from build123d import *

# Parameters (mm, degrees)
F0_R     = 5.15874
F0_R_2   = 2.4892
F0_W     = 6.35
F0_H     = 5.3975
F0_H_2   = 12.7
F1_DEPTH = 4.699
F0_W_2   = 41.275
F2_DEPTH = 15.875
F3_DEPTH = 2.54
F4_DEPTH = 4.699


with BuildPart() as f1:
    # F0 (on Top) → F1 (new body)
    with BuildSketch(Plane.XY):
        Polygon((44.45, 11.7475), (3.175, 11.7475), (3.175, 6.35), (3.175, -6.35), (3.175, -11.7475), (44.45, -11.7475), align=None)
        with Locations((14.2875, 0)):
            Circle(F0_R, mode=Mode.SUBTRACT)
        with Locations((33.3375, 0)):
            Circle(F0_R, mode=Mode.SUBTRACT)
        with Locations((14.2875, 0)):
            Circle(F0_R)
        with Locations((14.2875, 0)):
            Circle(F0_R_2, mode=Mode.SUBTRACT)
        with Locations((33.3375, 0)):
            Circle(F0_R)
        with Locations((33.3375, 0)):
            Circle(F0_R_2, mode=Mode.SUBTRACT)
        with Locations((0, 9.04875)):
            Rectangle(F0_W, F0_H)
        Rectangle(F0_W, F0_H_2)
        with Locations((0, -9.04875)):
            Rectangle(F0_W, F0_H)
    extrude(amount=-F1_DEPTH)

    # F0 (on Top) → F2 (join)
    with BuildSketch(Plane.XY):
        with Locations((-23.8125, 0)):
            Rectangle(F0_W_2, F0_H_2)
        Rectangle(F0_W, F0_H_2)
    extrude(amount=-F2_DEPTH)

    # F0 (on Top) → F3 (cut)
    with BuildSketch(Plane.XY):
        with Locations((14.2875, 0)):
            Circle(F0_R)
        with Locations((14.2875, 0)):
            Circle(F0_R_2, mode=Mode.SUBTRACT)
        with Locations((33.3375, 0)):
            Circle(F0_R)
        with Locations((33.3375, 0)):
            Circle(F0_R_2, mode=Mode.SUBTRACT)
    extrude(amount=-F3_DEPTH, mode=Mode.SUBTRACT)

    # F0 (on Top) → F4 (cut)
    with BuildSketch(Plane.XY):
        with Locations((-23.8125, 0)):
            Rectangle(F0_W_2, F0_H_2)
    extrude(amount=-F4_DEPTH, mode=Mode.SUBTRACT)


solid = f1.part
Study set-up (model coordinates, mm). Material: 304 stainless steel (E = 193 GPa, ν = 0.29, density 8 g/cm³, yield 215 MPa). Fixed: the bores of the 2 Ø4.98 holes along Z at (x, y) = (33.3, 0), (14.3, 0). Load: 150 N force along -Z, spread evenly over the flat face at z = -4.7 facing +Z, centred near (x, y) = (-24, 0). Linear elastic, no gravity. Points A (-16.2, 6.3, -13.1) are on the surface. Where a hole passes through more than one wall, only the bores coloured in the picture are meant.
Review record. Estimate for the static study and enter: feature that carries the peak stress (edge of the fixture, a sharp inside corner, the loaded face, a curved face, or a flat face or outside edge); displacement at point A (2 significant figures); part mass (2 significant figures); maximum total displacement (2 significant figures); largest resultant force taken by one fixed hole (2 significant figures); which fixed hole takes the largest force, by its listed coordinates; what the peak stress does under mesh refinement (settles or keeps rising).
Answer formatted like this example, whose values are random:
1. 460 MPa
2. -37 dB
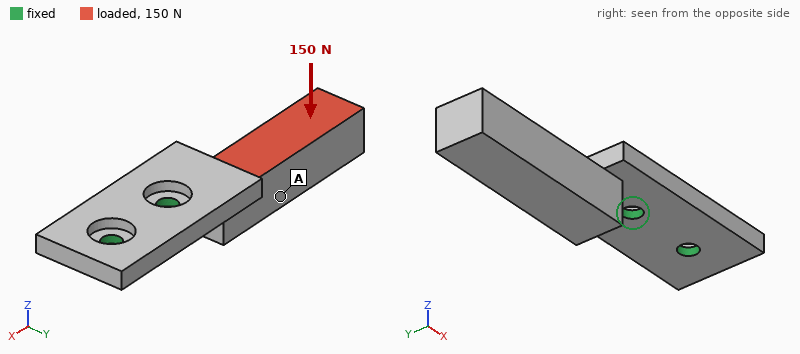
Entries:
1. edge of the fixture
2. 0.072 mm
3. 92 g
4. 0.15 mm
5. 550 N
6. (14.3, 0)
7. keeps rising
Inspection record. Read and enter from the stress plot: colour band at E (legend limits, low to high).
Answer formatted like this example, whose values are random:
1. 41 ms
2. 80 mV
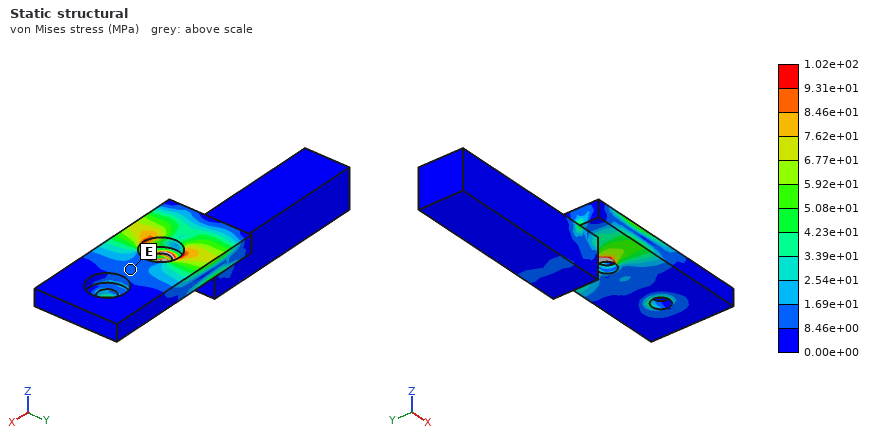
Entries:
1. 8.46e+00 to 1.69e+01 MPa
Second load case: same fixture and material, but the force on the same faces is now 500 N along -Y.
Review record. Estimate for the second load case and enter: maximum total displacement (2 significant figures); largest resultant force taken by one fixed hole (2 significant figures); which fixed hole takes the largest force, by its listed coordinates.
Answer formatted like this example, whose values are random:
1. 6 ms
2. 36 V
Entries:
1. 71 µm
2. 1.3 kN
3. (14.3, 0)
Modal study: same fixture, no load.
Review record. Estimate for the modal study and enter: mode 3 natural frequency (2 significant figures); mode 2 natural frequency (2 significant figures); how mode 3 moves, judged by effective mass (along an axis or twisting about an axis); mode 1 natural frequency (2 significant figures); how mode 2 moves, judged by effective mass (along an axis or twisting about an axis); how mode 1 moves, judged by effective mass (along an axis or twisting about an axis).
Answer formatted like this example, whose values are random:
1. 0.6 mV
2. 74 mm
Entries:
1. 5000 Hz
2. 2300 Hz
3. twisting about X
4. 860 Hz
5. along Y
6. along Z
